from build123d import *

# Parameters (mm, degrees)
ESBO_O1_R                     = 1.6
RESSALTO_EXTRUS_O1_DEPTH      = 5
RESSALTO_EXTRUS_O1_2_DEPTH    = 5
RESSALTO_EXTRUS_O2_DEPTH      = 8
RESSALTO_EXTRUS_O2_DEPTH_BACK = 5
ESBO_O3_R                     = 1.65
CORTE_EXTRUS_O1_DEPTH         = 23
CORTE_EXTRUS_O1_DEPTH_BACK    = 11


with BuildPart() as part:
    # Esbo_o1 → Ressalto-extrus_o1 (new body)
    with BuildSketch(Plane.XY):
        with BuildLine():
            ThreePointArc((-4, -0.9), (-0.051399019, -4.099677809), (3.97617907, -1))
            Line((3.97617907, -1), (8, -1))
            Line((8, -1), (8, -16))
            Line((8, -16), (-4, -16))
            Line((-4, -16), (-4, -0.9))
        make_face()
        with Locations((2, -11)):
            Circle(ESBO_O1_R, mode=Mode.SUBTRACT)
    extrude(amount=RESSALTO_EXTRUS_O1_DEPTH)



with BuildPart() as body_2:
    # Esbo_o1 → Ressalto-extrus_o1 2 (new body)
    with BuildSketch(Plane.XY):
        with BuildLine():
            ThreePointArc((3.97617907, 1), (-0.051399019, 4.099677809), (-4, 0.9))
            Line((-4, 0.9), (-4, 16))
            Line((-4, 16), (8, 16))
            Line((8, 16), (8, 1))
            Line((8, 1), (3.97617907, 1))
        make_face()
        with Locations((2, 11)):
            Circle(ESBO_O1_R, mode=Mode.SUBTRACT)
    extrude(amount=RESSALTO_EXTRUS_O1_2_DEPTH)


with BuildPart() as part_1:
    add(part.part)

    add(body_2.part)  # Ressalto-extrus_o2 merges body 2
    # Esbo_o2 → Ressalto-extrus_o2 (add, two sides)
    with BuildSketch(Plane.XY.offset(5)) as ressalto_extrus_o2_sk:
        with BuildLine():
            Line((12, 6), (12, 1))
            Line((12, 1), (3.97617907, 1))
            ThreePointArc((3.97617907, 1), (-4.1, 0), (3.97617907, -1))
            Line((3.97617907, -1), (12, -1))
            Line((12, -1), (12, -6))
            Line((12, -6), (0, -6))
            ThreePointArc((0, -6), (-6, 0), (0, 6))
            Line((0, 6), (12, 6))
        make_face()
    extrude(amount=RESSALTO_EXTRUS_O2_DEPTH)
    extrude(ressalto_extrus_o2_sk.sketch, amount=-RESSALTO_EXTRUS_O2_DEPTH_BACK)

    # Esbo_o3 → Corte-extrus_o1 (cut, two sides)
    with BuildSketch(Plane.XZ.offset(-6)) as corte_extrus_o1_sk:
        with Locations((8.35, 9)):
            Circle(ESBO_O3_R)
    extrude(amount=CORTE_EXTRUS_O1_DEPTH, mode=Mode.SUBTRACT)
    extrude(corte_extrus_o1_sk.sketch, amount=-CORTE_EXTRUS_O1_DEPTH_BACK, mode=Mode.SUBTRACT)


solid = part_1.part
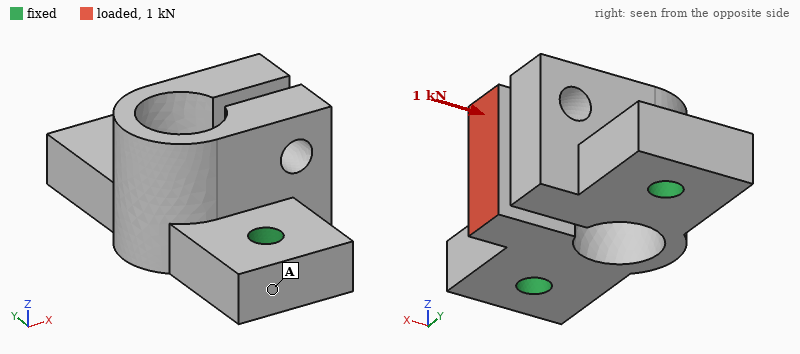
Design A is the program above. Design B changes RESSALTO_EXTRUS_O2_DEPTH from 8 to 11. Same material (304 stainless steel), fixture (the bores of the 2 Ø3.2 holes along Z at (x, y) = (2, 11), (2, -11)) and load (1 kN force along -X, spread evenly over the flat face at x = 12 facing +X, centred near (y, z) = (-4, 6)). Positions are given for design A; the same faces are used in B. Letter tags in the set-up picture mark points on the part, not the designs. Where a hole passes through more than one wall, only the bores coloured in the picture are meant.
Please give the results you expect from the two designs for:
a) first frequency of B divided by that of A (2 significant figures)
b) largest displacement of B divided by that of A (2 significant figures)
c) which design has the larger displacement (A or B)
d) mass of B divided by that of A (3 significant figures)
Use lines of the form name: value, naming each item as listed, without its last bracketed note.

first frequency of B divided by that of A: 0.76
largest displacement of B divided by that of A: 1.3
which design has the larger displacement: B
mass of B divided by that of A: 1.14
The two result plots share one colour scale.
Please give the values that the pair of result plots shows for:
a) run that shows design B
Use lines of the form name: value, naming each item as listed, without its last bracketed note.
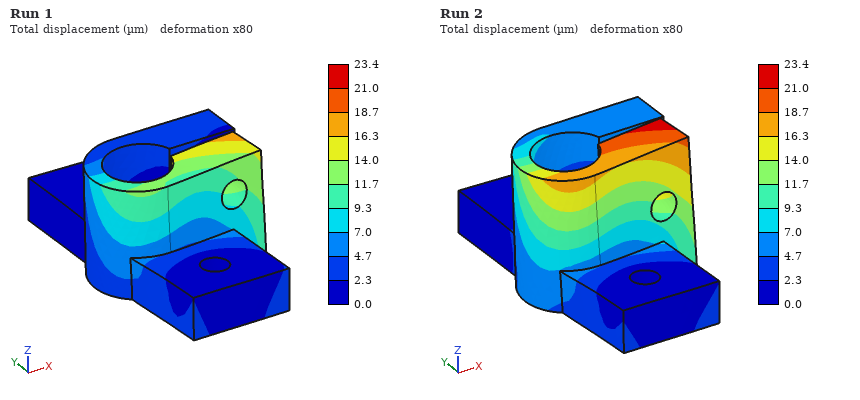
run that shows design B: Run 2
